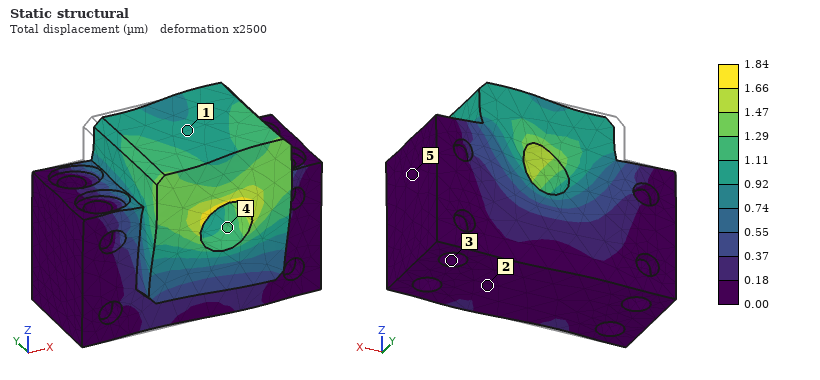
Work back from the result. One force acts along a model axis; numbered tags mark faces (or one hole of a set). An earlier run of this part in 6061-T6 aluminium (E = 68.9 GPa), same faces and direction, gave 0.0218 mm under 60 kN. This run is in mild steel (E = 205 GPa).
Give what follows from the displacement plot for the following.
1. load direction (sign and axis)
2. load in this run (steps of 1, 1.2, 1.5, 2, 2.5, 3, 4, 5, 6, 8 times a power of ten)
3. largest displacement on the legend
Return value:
+X
15 kN
1.84 µm
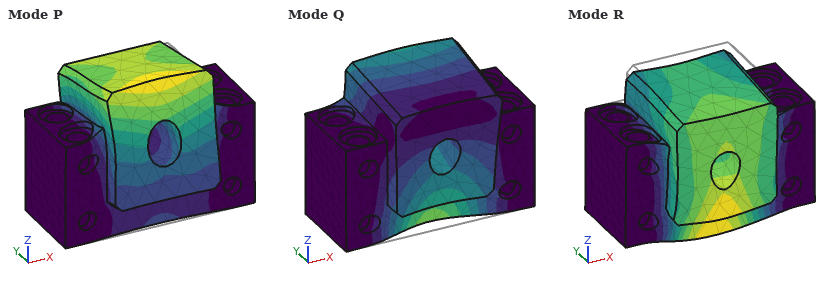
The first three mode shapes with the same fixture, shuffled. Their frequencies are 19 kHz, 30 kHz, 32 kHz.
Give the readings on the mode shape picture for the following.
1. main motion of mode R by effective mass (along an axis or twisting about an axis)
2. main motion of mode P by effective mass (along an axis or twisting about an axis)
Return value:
along Z
along Y
